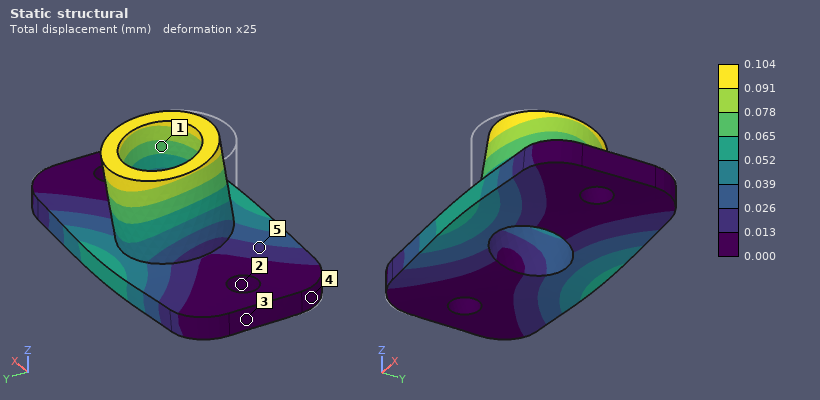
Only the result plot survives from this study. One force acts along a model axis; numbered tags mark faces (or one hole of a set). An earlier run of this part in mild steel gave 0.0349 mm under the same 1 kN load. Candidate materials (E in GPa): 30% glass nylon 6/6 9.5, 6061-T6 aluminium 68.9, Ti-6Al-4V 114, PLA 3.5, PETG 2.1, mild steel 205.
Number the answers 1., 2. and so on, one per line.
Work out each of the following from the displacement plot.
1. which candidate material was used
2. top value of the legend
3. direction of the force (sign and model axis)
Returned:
1. 6061-T6 aluminium
2. 0.104 mm
3. +Y
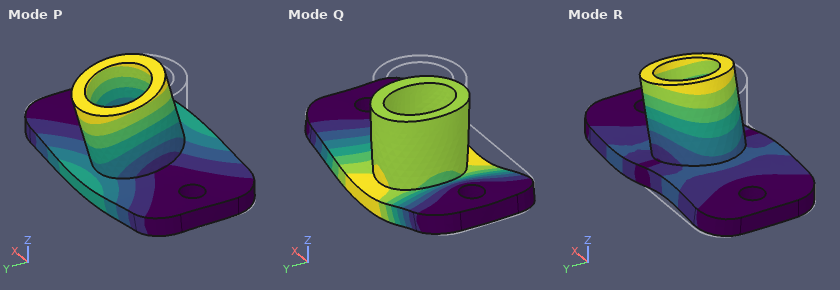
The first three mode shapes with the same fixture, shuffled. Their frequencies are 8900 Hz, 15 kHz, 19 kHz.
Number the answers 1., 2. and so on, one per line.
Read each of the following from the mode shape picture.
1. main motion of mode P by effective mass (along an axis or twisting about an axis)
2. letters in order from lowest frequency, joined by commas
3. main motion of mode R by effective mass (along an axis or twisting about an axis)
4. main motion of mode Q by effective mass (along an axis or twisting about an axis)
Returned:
1. along Y
2. P, Q, R
3. along X
4. along Z
